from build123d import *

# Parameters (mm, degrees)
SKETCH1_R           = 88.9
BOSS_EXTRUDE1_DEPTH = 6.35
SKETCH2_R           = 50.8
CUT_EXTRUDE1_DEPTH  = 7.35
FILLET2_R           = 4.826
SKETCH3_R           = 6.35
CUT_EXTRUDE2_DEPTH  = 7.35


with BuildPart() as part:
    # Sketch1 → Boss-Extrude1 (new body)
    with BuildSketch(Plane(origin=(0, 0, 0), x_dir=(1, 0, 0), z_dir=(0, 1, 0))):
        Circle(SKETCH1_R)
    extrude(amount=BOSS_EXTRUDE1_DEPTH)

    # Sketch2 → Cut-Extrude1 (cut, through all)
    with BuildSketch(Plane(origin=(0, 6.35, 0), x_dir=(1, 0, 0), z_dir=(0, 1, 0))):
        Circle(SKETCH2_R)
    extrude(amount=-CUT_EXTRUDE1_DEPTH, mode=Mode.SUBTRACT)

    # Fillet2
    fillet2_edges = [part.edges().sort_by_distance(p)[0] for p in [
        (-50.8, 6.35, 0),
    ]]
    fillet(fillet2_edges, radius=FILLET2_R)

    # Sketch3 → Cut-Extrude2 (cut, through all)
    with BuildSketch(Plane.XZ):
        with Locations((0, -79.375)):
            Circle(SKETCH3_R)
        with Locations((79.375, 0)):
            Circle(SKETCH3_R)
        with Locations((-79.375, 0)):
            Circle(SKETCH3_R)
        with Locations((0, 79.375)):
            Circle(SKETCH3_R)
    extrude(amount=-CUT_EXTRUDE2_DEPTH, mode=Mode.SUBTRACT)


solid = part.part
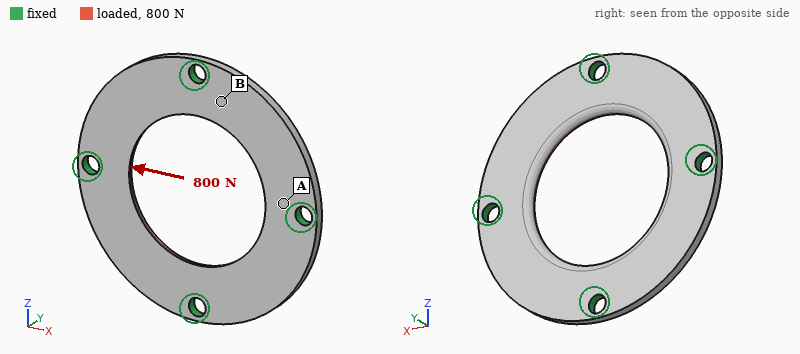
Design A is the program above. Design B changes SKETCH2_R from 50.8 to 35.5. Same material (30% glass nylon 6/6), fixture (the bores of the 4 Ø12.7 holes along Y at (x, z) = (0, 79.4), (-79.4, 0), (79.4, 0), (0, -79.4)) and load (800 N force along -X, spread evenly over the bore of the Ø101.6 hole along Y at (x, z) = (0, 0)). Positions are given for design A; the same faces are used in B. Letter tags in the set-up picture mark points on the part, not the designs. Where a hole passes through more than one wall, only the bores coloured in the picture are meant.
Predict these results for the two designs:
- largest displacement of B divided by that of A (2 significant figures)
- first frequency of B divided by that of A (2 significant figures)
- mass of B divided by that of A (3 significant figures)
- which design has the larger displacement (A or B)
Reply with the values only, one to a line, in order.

0.75
1.0
1.26
A
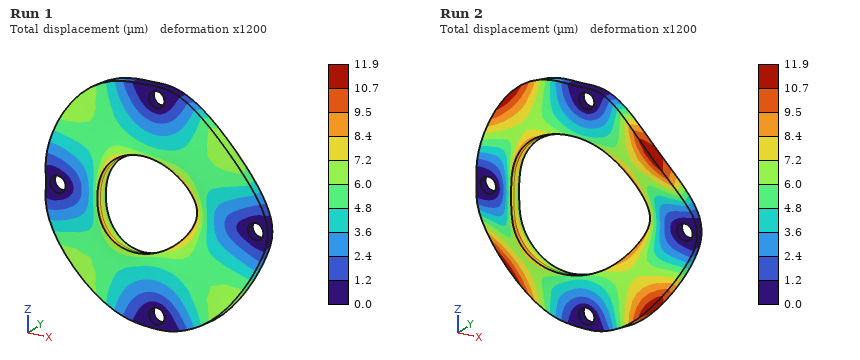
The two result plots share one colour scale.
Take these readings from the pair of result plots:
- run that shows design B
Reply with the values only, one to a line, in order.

Run 1
